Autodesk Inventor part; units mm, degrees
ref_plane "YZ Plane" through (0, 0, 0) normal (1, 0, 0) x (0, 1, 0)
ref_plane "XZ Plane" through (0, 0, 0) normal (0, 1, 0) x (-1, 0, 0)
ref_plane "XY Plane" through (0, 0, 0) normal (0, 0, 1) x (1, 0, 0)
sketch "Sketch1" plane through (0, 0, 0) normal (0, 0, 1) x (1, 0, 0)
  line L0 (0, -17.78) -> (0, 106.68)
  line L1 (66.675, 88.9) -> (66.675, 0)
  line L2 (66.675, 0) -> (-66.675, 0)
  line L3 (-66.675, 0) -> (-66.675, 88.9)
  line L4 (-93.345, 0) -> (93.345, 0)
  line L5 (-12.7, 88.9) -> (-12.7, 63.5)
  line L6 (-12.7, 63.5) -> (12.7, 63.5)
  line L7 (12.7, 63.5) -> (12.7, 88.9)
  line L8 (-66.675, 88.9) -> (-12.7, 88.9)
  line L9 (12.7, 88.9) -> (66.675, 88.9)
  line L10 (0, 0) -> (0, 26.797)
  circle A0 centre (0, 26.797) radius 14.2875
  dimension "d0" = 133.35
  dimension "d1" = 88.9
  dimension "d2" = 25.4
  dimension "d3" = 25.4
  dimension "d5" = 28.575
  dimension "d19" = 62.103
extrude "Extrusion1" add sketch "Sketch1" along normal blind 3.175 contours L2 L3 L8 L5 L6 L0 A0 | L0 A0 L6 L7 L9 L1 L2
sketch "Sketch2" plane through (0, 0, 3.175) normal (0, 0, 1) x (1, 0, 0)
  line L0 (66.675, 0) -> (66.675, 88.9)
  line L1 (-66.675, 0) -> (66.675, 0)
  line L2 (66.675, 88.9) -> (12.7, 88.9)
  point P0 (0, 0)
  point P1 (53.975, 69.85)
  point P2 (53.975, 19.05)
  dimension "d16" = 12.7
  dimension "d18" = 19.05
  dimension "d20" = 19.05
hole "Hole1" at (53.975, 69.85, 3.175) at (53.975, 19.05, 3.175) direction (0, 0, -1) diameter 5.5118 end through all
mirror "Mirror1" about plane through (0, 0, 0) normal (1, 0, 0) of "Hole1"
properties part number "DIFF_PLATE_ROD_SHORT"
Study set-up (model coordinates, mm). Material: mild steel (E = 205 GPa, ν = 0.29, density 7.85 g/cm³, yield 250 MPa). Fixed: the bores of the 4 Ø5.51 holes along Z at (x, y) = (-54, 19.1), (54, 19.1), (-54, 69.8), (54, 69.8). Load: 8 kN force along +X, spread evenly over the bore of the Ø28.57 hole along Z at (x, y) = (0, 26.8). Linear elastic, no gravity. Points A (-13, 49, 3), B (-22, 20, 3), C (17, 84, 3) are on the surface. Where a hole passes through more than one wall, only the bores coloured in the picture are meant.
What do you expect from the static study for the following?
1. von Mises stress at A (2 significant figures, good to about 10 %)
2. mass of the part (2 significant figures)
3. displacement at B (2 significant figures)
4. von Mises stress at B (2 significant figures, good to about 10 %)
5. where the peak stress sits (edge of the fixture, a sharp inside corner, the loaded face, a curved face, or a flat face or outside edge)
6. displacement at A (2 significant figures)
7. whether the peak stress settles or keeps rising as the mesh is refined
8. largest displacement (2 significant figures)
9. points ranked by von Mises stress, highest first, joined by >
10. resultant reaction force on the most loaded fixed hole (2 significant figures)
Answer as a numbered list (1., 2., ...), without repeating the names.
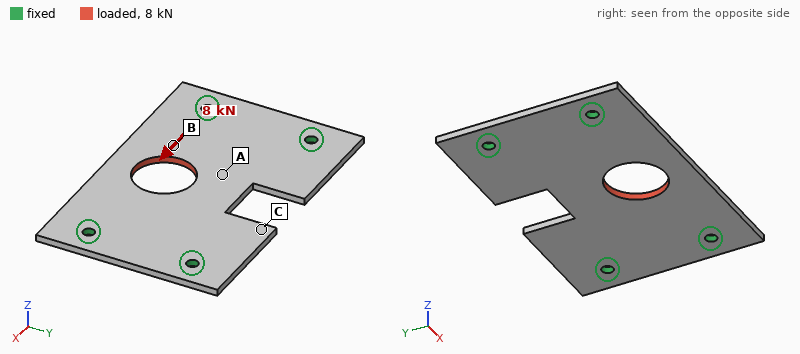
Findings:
1. 17 MPa
2. 260 g
3. 5.5 µm
4. 32 MPa
5. edge of the fixture
6. 3.9 µm
7. keeps rising
8. 8.2 µm
9. B > A > C
10. 2.8 kN
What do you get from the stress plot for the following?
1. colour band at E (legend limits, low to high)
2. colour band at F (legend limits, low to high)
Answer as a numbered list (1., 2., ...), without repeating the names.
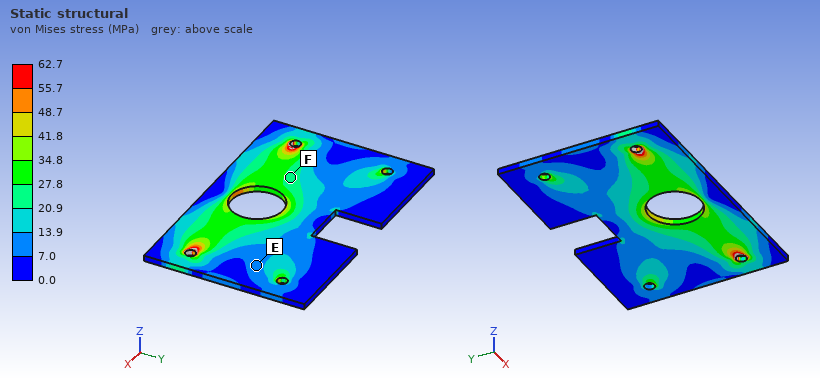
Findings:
1. 7.0 to 13.9 MPa
2. 20.9 to 27.8 MPa
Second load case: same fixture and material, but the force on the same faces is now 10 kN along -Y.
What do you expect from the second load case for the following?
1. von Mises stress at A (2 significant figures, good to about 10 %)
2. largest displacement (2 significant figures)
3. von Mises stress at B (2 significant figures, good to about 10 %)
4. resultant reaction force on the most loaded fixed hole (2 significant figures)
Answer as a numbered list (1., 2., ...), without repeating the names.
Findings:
1. 39 MPa
2. 26 µm
3. 50 MPa
4. 3.8 kN
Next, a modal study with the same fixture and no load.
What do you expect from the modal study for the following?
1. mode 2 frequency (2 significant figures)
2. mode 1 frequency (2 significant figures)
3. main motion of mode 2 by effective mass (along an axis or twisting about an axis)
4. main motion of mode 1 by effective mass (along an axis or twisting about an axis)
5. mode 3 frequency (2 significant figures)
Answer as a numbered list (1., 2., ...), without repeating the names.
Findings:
1. 1900 Hz
2. 1400 Hz
3. twisting about X
4. along Z
5. 2800 Hz
